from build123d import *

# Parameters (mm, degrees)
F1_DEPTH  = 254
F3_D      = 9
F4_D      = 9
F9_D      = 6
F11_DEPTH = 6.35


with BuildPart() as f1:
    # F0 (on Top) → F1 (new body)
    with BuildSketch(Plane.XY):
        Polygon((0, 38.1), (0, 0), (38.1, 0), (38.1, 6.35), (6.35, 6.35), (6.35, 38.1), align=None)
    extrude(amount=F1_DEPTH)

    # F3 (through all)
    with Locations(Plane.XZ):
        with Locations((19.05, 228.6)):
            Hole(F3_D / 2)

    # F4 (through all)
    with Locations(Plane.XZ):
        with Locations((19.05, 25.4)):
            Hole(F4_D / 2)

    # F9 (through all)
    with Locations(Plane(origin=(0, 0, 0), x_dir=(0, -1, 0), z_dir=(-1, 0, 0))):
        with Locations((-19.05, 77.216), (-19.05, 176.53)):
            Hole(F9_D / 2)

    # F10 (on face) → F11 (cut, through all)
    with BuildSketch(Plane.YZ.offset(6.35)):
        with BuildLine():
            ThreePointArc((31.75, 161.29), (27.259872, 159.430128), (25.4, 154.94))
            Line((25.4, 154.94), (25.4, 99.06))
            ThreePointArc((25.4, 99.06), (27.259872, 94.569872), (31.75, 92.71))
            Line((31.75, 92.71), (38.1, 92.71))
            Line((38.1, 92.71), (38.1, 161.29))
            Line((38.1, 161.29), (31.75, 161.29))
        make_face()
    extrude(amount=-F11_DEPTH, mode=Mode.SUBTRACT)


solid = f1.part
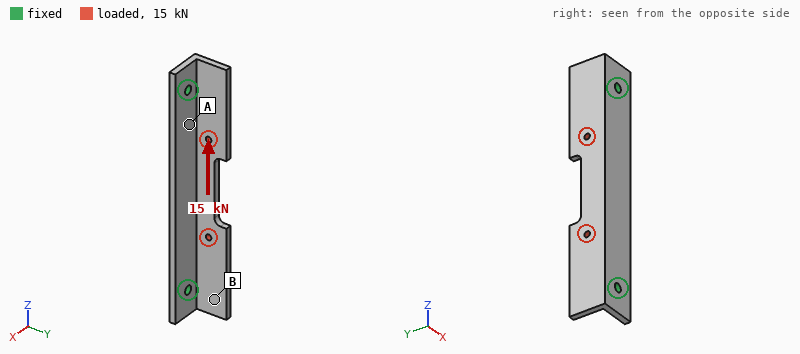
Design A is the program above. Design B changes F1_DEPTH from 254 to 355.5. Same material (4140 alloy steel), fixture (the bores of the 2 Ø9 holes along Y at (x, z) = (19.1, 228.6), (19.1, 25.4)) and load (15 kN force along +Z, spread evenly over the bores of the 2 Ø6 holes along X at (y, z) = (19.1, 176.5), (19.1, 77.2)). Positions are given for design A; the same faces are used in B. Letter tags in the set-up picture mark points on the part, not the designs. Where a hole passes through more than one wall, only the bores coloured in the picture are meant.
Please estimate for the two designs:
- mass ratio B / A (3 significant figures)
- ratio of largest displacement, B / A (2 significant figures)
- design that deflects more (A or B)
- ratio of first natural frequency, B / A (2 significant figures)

1.42
1.8
B
0.55
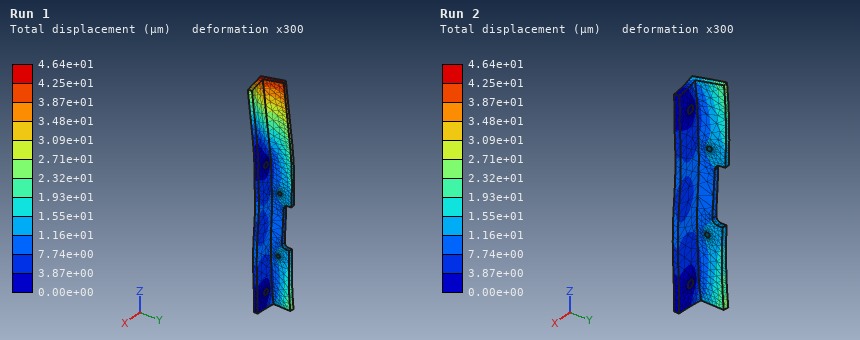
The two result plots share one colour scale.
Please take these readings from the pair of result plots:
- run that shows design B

Run 1
